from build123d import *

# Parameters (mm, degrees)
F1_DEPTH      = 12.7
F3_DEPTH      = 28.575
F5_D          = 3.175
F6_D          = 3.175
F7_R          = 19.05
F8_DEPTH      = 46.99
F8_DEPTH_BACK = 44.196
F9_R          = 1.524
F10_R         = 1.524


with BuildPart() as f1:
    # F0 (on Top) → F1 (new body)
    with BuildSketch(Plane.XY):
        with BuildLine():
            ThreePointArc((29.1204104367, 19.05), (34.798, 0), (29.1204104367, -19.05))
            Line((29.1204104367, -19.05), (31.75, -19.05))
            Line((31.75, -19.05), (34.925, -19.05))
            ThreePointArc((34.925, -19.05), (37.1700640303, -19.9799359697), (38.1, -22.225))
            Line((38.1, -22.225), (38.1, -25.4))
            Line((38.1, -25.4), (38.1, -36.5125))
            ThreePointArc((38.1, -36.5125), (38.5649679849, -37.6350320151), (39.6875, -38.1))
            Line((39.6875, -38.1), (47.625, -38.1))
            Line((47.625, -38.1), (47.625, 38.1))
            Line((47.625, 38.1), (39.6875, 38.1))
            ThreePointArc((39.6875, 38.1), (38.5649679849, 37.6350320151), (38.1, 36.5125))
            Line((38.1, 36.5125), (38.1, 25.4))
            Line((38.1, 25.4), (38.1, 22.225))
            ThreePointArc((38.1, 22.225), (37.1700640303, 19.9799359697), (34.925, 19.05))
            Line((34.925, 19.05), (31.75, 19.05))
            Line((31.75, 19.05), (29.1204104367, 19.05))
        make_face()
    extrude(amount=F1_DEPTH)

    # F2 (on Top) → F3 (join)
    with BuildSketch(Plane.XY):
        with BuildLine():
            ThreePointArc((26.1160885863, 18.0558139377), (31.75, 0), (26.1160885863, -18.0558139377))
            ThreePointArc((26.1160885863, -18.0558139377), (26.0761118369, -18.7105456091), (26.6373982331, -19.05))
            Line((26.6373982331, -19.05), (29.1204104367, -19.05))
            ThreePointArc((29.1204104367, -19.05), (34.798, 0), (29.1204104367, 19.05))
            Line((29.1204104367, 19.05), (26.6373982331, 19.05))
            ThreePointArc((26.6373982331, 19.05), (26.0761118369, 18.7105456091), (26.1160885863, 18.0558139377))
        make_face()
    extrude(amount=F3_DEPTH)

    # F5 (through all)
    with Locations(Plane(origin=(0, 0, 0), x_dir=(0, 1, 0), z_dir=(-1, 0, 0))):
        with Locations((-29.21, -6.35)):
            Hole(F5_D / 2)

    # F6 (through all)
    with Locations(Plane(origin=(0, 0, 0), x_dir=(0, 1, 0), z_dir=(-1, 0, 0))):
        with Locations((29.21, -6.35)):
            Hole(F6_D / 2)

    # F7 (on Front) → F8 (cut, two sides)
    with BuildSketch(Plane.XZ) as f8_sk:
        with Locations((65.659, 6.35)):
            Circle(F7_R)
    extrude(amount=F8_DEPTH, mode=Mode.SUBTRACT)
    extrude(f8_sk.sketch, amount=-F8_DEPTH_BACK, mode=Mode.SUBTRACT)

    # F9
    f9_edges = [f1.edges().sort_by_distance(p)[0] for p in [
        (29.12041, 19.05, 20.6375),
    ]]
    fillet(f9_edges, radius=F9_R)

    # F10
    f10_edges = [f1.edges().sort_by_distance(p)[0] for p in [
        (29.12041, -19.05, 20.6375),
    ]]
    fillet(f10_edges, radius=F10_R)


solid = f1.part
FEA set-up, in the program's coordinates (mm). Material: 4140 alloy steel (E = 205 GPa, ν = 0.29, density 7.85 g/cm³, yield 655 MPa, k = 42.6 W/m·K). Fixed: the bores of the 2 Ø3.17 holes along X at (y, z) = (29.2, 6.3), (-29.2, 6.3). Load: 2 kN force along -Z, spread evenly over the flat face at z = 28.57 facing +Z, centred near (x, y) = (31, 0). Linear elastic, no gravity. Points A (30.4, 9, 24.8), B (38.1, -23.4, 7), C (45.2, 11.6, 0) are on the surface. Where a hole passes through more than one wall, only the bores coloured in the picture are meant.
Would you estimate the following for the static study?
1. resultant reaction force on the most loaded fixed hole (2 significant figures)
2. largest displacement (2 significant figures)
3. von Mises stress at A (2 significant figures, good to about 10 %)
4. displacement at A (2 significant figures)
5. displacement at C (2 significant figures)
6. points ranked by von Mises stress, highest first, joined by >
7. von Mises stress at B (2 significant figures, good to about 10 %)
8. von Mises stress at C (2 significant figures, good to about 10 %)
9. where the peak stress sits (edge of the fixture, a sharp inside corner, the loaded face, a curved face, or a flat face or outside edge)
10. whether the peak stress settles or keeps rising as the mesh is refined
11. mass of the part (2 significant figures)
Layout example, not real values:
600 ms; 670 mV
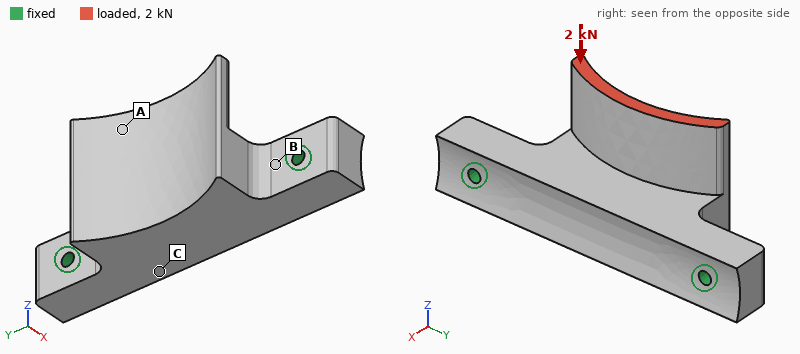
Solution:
1.0 kN; 35 µm; 15 MPa; 28 µm; 7.1 µm; B > C > A; 99 MPa; 24 MPa; edge of the fixture; keeps rising; 110 g
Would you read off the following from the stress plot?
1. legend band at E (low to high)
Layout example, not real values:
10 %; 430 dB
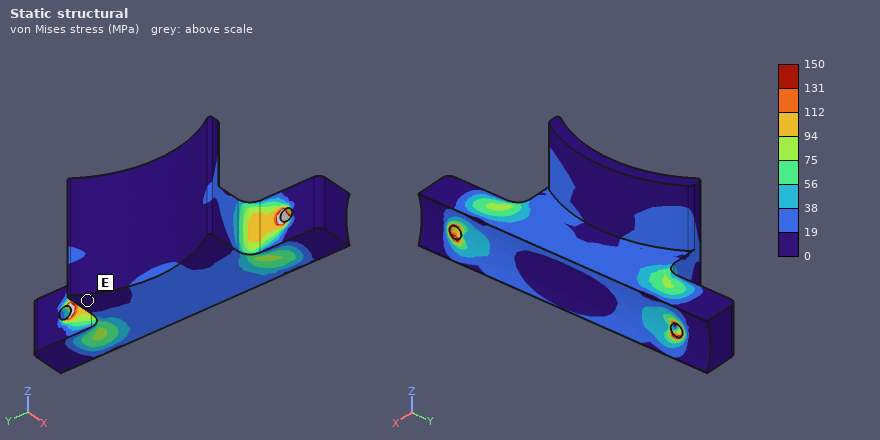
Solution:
0 to 19 MPa
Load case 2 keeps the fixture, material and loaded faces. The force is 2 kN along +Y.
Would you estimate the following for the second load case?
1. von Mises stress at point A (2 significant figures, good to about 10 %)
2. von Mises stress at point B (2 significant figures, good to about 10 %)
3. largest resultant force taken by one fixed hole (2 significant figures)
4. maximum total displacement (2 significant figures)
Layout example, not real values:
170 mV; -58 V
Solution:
93 MPa; 47 MPa; 1.4 kN; 39 µm
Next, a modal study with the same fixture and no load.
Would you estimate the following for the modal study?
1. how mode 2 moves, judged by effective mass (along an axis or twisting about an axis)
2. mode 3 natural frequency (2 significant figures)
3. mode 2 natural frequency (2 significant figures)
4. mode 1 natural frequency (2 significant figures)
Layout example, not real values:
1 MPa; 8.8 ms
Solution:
along Z; 11 kHz; 9100 Hz; 6400 Hz
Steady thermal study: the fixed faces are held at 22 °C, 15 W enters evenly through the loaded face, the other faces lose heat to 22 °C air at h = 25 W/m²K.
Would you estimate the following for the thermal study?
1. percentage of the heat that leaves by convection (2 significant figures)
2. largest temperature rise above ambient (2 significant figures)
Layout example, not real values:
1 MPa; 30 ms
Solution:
21 %; 72 K
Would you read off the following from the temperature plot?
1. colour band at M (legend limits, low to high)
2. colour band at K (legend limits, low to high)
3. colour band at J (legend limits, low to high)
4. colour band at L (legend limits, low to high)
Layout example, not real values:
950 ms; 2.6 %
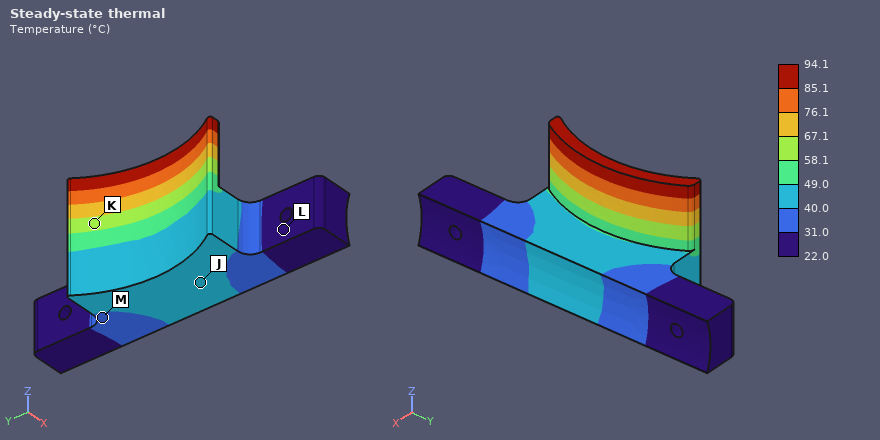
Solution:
31.0 to 40.0 °C; 58.1 to 67.1 °C; 40.0 to 49.0 °C; 22.0 to 31.0 °C
